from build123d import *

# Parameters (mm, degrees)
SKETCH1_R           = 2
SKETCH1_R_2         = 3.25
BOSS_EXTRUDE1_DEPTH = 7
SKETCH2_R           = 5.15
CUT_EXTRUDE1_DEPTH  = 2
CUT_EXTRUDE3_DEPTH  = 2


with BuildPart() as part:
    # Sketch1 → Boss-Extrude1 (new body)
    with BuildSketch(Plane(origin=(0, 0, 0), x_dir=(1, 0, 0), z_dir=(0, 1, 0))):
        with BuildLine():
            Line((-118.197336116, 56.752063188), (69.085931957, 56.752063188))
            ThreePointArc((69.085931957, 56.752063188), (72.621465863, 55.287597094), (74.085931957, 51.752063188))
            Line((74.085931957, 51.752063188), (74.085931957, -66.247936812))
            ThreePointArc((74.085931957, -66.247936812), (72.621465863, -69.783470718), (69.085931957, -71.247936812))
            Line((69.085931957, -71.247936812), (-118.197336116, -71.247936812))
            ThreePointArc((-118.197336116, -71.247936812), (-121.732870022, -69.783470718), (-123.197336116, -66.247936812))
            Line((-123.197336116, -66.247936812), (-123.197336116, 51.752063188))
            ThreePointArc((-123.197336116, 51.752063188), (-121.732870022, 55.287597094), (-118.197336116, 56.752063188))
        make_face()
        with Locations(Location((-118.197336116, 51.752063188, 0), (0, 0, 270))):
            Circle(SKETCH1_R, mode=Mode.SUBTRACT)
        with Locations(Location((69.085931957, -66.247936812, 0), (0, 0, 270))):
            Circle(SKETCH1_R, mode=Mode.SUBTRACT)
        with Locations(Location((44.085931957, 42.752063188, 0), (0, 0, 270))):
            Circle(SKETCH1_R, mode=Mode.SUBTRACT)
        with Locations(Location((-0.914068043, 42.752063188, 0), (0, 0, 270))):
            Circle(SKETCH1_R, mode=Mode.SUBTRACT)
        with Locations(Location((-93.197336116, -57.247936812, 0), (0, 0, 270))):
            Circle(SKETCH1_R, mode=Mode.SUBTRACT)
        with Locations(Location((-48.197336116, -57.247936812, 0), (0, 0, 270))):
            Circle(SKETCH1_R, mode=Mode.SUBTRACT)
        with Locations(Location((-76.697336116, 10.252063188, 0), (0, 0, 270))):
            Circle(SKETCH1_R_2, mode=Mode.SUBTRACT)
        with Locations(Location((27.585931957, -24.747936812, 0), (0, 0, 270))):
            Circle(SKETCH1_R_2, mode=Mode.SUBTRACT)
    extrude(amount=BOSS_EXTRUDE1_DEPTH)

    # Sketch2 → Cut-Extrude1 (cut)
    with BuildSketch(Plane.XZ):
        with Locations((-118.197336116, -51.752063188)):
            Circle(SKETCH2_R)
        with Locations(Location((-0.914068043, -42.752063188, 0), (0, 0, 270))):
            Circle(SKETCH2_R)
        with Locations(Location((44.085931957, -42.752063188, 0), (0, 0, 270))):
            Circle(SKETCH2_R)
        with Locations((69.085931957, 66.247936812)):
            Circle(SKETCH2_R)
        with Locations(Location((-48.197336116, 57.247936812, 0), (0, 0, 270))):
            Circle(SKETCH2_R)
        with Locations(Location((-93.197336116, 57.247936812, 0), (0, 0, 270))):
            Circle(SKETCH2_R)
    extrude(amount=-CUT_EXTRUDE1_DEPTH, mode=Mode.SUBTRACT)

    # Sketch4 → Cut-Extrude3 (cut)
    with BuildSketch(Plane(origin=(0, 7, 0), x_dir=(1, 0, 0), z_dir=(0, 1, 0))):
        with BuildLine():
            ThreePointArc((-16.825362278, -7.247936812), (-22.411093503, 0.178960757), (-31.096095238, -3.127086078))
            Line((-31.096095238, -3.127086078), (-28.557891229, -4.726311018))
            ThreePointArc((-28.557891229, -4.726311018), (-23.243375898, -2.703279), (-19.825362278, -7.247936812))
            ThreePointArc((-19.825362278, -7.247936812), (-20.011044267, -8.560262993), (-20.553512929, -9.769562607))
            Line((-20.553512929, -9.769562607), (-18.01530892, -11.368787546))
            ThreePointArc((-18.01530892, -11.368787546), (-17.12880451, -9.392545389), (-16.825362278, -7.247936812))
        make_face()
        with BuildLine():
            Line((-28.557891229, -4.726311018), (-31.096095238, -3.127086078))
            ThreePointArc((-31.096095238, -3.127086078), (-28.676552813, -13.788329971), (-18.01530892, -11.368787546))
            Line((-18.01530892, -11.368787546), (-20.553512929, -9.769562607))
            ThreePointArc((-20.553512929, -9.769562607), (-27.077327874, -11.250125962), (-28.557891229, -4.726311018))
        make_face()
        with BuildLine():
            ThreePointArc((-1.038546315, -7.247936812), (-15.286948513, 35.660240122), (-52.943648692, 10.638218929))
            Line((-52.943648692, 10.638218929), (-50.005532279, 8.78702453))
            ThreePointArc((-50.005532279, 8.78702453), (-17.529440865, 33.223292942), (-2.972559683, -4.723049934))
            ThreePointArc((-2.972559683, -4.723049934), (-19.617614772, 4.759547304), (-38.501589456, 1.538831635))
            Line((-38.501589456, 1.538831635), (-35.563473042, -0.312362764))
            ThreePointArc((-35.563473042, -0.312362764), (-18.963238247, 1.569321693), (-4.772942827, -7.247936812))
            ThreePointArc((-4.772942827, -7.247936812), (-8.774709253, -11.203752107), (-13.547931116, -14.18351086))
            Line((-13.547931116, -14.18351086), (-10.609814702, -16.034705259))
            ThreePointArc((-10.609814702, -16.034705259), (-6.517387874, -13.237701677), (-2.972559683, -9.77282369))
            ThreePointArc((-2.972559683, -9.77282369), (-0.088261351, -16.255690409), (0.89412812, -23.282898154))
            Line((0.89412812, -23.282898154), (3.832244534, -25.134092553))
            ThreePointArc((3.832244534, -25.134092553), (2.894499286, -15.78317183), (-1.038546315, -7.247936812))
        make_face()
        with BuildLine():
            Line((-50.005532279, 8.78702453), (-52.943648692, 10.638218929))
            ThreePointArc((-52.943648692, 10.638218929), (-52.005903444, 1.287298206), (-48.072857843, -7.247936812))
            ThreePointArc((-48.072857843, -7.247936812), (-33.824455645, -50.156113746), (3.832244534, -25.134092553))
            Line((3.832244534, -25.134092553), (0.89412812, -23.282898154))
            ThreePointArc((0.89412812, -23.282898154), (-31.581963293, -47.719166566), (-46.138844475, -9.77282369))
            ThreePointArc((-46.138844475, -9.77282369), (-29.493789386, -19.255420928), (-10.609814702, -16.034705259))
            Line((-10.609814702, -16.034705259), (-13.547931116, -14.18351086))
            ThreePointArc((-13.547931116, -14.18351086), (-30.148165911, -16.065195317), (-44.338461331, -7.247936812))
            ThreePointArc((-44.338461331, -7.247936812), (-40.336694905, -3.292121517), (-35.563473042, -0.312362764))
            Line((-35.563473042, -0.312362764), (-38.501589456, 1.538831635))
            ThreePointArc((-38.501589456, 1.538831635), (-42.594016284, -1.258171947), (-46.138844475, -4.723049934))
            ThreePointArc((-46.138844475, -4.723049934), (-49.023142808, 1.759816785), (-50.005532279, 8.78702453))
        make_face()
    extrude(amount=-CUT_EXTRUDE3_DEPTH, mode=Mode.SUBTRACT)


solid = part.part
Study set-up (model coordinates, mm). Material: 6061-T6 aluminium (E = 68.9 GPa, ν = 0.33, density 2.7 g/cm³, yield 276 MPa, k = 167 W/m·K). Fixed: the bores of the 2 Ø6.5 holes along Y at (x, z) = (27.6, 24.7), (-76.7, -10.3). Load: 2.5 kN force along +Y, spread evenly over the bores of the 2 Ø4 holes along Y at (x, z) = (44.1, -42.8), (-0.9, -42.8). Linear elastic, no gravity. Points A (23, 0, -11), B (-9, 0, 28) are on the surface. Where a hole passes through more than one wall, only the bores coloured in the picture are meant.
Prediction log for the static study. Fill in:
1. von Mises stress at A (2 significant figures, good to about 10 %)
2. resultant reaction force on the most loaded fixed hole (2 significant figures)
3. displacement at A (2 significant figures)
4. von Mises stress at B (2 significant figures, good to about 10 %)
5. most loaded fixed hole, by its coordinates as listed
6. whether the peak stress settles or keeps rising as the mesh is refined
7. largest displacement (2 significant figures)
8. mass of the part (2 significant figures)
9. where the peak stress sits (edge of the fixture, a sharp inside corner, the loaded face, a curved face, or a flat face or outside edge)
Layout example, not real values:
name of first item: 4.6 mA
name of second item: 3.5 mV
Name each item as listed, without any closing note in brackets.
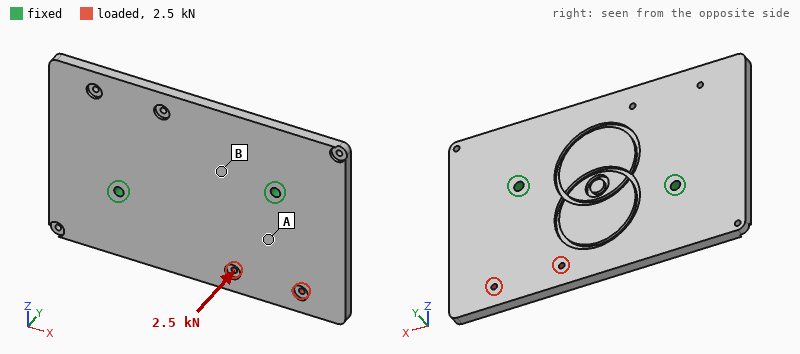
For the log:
von Mises stress at A: 65 MPa
resultant reaction force on the most loaded fixed hole: 1.9 kN
displacement at A: 0.48 mm
von Mises stress at B: 26 MPa
most loaded fixed hole, by its coordinates as listed: (27.6, 24.7)
whether the peak stress settles or keeps rising as the mesh is refined: keeps rising
largest displacement: 1.8 mm
mass of the part: 470 g
where the peak stress sits: edge of the fixture
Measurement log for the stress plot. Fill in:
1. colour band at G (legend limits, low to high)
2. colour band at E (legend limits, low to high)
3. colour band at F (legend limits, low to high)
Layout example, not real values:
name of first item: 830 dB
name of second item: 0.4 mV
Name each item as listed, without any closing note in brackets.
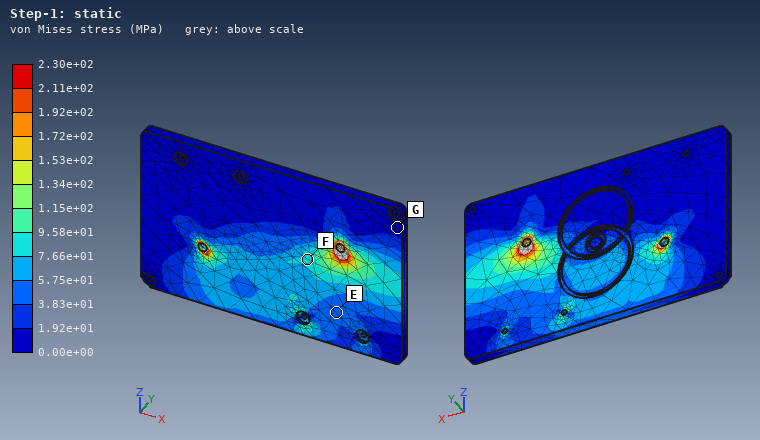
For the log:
colour band at G: 0.00e+00 to 1.92e+01 MPa
colour band at E: 3.83e+01 to 5.75e+01 MPa
colour band at F: 7.66e+01 to 9.58e+01 MPa
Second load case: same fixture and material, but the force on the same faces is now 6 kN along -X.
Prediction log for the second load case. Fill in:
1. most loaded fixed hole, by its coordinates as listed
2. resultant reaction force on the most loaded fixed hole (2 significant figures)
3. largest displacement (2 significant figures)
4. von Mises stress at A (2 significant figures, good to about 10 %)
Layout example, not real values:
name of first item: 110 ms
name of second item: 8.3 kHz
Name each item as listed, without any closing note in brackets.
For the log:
most loaded fixed hole, by its coordinates as listed: (-76.7, -10.3)
resultant reaction force on the most loaded fixed hole: 4.6 kN
largest displacement: 89 µm
von Mises stress at A: 5.9 MPa
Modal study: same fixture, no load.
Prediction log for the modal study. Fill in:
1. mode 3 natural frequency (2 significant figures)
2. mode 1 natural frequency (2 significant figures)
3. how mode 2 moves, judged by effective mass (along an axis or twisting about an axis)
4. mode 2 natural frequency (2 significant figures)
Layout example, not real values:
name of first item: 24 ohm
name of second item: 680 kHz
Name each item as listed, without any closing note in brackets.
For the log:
mode 3 natural frequency: 1500 Hz
mode 1 natural frequency: 760 Hz
how mode 2 moves, judged by effective mass: along Y
mode 2 natural frequency: 960 Hz
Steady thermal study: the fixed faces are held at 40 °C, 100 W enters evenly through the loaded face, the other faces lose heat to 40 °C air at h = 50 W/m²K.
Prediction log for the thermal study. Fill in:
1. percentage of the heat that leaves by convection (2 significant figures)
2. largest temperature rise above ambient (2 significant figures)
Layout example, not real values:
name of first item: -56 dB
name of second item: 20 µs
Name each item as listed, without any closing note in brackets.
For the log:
percentage of the heat that leaves by convection: 38 %
largest temperature rise above ambient: 61 K
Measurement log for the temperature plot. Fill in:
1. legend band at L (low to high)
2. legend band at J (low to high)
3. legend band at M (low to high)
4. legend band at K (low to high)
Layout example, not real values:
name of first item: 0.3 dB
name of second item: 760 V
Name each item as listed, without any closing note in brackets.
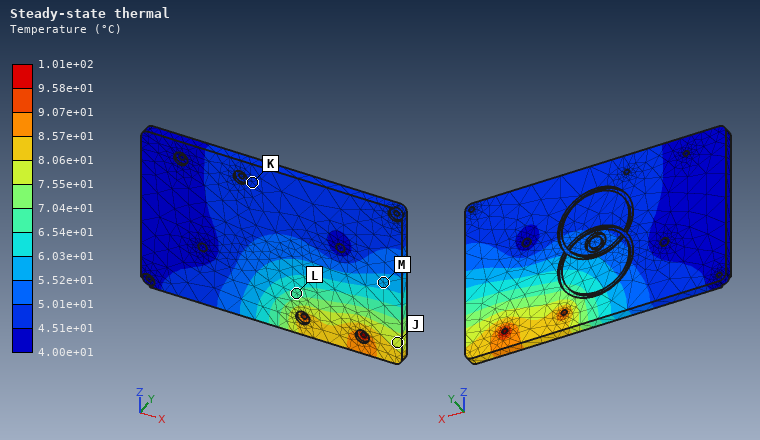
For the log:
legend band at L: 6.54e+01 to 7.04e+01 °C
legend band at J: 7.55e+01 to 8.06e+01 °C
legend band at M: 5.52e+01 to 6.03e+01 °C
legend band at K: 4.51e+01 to 5.01e+01 °C
